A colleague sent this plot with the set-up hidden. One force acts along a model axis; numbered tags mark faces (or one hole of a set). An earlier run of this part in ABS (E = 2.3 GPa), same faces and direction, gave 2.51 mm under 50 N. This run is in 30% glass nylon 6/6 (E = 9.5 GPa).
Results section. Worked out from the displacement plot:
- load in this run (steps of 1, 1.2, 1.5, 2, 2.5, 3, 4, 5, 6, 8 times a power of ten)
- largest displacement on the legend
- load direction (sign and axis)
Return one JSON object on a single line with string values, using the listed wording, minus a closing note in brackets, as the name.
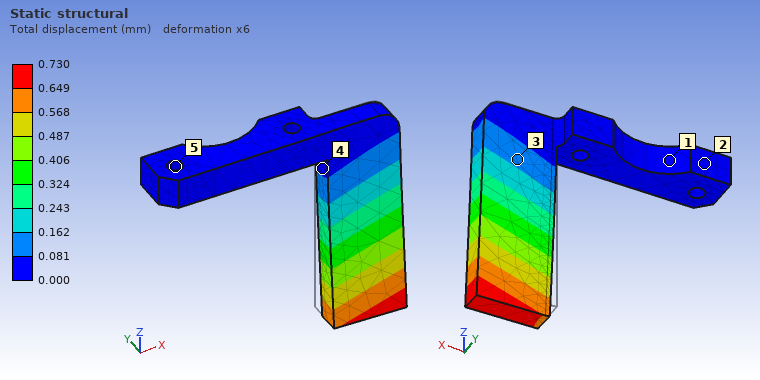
{"load in this run": "60 N", "largest displacement on the legend": "0.730 mm", "load direction": "-Y"}
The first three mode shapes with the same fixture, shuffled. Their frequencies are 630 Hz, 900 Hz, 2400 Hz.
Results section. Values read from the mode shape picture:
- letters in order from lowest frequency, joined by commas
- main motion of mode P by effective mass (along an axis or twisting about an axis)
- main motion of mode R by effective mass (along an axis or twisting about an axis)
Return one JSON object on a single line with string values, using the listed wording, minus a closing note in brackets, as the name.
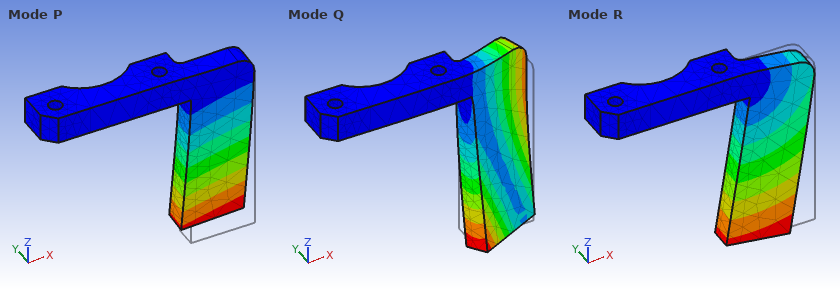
{"letters in order from lowest frequency, joined by commas": "P, R, Q", "main motion of mode P by effective mass": "along Y", "main motion of mode R by effective mass": "along X"}
